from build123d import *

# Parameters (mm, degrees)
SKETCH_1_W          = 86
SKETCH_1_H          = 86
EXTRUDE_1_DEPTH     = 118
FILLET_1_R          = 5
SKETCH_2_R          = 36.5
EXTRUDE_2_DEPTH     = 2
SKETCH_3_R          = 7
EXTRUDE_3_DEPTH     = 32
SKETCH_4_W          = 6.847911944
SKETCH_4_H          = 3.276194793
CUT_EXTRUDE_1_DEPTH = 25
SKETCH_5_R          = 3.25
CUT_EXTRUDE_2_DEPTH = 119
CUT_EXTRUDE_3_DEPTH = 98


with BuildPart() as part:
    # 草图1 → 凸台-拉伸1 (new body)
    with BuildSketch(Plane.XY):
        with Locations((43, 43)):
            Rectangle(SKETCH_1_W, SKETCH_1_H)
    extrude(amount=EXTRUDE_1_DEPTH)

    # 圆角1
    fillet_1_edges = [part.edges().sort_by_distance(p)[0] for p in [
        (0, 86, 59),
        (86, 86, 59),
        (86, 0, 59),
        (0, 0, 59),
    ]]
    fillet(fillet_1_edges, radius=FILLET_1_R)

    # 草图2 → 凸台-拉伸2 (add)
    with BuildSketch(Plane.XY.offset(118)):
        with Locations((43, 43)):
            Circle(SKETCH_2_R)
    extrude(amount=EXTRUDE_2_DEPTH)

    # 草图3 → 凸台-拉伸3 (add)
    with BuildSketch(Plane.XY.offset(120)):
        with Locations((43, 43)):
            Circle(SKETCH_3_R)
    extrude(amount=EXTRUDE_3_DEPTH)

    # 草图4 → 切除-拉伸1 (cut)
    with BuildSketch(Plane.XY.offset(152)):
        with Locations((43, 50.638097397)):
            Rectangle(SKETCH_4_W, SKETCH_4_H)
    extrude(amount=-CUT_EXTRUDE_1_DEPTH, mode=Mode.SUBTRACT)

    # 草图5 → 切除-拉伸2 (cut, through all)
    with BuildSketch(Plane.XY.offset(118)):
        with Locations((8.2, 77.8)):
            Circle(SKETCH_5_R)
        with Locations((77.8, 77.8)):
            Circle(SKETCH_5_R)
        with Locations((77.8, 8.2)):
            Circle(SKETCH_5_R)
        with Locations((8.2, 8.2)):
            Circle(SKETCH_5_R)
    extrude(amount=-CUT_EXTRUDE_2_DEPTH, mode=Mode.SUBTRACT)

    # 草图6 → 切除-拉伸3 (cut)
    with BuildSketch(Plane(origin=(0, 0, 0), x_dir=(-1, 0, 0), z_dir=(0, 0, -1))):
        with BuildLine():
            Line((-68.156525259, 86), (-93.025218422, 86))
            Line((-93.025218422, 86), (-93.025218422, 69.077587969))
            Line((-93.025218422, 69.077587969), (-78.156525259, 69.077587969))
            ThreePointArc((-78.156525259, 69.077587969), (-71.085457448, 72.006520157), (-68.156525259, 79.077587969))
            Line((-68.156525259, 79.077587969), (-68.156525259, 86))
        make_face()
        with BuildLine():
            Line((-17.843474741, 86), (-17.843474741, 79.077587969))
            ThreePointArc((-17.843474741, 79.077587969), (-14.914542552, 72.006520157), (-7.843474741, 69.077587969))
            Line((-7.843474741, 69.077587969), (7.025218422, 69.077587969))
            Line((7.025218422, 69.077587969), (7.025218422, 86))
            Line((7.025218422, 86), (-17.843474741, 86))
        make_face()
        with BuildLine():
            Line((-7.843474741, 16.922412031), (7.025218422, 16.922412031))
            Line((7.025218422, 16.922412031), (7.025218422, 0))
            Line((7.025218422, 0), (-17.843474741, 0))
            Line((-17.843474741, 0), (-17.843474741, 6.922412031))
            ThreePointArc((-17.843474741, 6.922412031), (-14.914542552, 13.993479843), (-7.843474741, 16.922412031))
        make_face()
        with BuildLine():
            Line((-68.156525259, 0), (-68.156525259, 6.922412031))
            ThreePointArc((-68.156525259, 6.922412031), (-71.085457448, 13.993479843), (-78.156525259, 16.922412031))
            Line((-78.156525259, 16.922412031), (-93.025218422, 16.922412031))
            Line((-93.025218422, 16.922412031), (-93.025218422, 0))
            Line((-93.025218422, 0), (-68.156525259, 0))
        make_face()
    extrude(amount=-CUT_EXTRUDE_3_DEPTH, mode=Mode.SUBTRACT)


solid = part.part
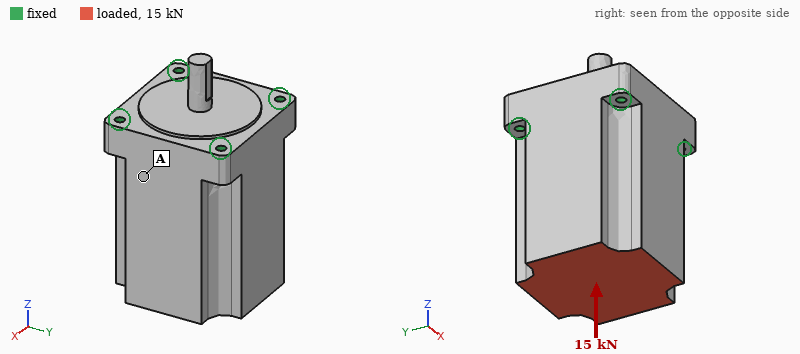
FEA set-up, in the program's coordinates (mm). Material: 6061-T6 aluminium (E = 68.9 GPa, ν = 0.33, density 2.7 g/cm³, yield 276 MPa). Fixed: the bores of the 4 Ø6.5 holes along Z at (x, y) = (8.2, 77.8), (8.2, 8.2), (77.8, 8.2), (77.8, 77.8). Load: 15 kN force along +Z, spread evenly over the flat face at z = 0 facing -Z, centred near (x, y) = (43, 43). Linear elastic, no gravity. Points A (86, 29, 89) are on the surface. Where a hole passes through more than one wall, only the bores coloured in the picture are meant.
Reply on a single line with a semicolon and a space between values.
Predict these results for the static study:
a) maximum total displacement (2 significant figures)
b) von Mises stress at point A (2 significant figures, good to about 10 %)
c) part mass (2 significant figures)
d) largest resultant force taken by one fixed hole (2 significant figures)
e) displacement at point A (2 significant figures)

8.1 µm; 3.8 MPa; 2.1 kg; 3.9 kN; 4.8 µm
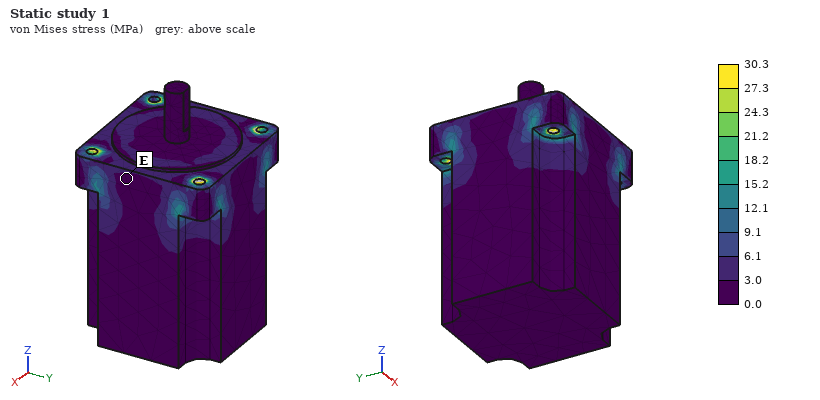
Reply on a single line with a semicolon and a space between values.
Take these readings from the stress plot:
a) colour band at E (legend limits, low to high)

0.0 to 3.0 MPa
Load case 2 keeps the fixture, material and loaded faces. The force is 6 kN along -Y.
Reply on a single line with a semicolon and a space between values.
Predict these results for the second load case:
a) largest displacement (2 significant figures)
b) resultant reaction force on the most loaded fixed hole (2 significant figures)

35 µm; 5.1 kN
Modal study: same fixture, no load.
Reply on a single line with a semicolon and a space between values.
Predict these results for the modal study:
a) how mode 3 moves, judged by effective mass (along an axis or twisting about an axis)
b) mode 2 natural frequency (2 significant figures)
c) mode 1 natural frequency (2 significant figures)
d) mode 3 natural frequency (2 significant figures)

along Z; 2700 Hz; 2700 Hz; 5800 Hz
